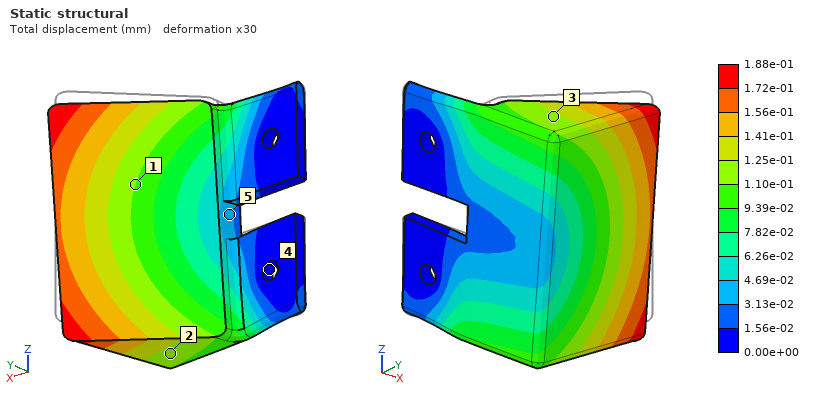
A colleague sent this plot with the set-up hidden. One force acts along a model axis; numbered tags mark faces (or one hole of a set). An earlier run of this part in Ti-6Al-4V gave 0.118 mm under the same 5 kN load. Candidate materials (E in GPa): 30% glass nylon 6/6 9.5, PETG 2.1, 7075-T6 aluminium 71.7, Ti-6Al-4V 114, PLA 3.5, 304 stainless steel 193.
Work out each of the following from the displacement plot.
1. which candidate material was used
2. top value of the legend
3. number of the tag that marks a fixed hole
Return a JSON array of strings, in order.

["7075-T6 aluminium", "1.88e-01 mm", "4"]
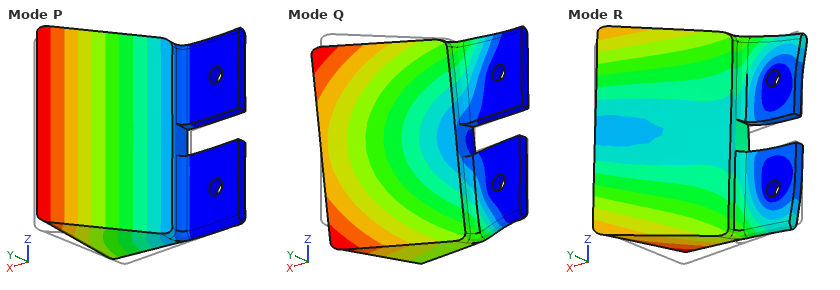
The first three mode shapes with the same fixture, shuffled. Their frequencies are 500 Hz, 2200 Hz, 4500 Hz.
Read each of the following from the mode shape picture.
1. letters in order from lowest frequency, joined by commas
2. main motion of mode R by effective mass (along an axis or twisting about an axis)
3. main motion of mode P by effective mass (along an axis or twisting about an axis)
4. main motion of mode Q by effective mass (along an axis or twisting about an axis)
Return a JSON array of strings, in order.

["P, Q, R", "along Z", "along Y", "along Z"]
